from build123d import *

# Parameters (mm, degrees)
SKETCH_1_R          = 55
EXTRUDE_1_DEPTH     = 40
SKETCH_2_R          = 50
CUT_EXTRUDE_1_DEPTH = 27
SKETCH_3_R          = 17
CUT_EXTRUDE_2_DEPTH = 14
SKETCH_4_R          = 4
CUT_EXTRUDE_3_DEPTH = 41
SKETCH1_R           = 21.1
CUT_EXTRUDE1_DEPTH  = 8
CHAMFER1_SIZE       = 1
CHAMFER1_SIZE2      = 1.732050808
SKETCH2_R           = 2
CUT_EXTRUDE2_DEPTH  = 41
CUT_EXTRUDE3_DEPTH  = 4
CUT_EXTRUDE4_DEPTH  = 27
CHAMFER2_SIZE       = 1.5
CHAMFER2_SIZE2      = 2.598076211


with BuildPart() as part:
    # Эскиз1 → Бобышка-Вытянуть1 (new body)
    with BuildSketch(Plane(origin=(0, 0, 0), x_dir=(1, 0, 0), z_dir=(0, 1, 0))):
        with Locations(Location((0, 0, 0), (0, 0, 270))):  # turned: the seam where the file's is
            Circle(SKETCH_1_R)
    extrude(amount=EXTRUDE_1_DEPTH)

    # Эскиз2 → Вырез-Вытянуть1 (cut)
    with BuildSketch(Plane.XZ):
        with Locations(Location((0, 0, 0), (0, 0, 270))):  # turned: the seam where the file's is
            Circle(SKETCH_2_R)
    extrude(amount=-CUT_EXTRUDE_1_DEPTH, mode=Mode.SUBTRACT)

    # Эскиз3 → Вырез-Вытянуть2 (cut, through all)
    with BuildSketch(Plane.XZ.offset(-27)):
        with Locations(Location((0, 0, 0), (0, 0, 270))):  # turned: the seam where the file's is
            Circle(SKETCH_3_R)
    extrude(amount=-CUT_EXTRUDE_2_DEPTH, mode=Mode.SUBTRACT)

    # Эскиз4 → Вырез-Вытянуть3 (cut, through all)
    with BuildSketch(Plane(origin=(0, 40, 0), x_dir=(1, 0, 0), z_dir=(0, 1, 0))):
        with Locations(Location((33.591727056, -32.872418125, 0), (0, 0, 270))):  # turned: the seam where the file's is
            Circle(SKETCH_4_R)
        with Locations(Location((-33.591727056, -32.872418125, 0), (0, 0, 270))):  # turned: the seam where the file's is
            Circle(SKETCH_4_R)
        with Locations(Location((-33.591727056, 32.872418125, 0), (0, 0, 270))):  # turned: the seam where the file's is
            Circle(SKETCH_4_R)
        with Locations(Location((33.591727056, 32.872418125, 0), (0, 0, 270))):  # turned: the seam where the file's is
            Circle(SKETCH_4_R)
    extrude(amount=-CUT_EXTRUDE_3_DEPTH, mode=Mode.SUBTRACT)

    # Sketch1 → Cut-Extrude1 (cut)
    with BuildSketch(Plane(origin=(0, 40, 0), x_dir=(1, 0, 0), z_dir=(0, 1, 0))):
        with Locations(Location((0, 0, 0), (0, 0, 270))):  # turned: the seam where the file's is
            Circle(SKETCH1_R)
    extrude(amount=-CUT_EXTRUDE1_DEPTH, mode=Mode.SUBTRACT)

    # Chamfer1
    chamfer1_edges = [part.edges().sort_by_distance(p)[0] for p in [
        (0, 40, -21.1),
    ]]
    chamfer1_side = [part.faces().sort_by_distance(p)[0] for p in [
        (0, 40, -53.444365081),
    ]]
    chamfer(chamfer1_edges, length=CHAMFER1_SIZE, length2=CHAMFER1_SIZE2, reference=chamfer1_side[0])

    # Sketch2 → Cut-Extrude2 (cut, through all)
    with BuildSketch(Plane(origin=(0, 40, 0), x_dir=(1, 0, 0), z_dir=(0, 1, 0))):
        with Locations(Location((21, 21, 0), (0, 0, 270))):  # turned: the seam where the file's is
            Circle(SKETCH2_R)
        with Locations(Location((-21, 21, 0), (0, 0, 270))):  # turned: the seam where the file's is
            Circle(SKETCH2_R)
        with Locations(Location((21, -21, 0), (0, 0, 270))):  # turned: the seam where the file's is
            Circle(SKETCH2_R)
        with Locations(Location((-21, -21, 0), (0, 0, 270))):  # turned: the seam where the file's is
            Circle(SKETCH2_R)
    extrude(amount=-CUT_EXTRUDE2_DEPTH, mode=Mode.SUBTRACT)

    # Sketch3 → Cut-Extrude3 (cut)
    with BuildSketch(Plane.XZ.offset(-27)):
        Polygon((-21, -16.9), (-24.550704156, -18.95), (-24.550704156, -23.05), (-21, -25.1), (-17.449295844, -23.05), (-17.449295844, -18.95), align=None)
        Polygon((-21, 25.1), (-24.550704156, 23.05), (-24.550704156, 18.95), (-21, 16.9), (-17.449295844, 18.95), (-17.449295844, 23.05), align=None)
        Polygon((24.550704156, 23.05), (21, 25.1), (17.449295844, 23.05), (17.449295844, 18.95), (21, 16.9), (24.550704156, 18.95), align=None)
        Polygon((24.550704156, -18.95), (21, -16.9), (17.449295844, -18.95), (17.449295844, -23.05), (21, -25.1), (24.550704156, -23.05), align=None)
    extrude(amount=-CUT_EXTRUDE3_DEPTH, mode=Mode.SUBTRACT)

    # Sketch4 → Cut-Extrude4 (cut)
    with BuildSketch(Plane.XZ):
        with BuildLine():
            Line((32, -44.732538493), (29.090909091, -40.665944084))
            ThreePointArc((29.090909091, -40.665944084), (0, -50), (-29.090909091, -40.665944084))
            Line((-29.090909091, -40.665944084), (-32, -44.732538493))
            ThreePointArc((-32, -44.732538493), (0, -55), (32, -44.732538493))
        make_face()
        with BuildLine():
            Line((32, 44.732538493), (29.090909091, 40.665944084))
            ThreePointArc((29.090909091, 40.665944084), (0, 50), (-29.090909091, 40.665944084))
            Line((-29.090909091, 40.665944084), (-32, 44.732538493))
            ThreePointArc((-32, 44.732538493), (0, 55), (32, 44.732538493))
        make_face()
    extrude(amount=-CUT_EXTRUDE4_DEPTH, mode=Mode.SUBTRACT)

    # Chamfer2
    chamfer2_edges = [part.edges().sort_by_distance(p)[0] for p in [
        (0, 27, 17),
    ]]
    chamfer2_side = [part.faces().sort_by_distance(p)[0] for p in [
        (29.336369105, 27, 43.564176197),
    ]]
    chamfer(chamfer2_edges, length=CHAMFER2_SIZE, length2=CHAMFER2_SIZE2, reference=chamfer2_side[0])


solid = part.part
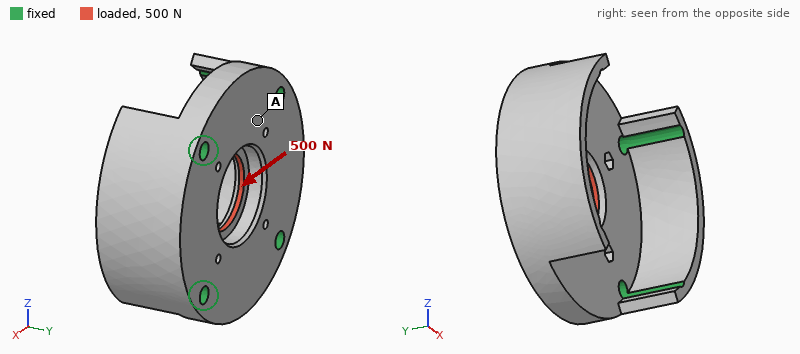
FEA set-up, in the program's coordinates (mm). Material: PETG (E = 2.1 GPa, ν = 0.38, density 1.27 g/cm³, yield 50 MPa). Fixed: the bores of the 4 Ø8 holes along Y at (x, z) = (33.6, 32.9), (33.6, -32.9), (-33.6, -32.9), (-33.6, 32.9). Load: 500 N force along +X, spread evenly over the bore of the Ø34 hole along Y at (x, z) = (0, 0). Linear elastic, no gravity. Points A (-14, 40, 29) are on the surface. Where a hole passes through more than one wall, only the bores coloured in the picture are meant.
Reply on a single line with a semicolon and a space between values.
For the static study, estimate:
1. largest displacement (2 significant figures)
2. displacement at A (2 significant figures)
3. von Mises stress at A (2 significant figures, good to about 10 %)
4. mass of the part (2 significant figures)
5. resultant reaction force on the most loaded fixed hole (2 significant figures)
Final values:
15 µm; 2.6 µm; 0.32 MPa; 170 g; 130 N
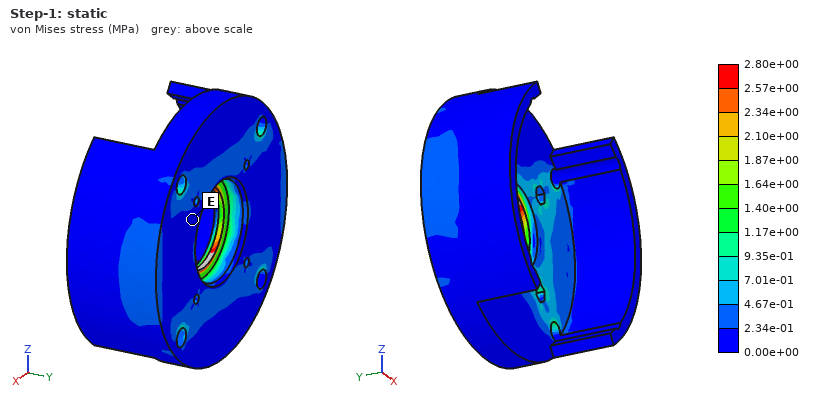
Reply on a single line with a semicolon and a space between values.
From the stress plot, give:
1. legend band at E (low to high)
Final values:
0.00e+00 to 2.34e-01 MPa
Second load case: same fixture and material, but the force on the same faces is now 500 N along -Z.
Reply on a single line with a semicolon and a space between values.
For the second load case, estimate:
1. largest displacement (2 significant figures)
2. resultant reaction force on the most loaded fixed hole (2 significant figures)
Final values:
16 µm; 130 N
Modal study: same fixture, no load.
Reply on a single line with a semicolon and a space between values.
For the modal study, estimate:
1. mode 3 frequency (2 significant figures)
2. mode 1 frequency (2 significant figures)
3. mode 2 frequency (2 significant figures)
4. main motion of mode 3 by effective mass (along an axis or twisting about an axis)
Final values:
3000 Hz; 2800 Hz; 2800 Hz; along Y
